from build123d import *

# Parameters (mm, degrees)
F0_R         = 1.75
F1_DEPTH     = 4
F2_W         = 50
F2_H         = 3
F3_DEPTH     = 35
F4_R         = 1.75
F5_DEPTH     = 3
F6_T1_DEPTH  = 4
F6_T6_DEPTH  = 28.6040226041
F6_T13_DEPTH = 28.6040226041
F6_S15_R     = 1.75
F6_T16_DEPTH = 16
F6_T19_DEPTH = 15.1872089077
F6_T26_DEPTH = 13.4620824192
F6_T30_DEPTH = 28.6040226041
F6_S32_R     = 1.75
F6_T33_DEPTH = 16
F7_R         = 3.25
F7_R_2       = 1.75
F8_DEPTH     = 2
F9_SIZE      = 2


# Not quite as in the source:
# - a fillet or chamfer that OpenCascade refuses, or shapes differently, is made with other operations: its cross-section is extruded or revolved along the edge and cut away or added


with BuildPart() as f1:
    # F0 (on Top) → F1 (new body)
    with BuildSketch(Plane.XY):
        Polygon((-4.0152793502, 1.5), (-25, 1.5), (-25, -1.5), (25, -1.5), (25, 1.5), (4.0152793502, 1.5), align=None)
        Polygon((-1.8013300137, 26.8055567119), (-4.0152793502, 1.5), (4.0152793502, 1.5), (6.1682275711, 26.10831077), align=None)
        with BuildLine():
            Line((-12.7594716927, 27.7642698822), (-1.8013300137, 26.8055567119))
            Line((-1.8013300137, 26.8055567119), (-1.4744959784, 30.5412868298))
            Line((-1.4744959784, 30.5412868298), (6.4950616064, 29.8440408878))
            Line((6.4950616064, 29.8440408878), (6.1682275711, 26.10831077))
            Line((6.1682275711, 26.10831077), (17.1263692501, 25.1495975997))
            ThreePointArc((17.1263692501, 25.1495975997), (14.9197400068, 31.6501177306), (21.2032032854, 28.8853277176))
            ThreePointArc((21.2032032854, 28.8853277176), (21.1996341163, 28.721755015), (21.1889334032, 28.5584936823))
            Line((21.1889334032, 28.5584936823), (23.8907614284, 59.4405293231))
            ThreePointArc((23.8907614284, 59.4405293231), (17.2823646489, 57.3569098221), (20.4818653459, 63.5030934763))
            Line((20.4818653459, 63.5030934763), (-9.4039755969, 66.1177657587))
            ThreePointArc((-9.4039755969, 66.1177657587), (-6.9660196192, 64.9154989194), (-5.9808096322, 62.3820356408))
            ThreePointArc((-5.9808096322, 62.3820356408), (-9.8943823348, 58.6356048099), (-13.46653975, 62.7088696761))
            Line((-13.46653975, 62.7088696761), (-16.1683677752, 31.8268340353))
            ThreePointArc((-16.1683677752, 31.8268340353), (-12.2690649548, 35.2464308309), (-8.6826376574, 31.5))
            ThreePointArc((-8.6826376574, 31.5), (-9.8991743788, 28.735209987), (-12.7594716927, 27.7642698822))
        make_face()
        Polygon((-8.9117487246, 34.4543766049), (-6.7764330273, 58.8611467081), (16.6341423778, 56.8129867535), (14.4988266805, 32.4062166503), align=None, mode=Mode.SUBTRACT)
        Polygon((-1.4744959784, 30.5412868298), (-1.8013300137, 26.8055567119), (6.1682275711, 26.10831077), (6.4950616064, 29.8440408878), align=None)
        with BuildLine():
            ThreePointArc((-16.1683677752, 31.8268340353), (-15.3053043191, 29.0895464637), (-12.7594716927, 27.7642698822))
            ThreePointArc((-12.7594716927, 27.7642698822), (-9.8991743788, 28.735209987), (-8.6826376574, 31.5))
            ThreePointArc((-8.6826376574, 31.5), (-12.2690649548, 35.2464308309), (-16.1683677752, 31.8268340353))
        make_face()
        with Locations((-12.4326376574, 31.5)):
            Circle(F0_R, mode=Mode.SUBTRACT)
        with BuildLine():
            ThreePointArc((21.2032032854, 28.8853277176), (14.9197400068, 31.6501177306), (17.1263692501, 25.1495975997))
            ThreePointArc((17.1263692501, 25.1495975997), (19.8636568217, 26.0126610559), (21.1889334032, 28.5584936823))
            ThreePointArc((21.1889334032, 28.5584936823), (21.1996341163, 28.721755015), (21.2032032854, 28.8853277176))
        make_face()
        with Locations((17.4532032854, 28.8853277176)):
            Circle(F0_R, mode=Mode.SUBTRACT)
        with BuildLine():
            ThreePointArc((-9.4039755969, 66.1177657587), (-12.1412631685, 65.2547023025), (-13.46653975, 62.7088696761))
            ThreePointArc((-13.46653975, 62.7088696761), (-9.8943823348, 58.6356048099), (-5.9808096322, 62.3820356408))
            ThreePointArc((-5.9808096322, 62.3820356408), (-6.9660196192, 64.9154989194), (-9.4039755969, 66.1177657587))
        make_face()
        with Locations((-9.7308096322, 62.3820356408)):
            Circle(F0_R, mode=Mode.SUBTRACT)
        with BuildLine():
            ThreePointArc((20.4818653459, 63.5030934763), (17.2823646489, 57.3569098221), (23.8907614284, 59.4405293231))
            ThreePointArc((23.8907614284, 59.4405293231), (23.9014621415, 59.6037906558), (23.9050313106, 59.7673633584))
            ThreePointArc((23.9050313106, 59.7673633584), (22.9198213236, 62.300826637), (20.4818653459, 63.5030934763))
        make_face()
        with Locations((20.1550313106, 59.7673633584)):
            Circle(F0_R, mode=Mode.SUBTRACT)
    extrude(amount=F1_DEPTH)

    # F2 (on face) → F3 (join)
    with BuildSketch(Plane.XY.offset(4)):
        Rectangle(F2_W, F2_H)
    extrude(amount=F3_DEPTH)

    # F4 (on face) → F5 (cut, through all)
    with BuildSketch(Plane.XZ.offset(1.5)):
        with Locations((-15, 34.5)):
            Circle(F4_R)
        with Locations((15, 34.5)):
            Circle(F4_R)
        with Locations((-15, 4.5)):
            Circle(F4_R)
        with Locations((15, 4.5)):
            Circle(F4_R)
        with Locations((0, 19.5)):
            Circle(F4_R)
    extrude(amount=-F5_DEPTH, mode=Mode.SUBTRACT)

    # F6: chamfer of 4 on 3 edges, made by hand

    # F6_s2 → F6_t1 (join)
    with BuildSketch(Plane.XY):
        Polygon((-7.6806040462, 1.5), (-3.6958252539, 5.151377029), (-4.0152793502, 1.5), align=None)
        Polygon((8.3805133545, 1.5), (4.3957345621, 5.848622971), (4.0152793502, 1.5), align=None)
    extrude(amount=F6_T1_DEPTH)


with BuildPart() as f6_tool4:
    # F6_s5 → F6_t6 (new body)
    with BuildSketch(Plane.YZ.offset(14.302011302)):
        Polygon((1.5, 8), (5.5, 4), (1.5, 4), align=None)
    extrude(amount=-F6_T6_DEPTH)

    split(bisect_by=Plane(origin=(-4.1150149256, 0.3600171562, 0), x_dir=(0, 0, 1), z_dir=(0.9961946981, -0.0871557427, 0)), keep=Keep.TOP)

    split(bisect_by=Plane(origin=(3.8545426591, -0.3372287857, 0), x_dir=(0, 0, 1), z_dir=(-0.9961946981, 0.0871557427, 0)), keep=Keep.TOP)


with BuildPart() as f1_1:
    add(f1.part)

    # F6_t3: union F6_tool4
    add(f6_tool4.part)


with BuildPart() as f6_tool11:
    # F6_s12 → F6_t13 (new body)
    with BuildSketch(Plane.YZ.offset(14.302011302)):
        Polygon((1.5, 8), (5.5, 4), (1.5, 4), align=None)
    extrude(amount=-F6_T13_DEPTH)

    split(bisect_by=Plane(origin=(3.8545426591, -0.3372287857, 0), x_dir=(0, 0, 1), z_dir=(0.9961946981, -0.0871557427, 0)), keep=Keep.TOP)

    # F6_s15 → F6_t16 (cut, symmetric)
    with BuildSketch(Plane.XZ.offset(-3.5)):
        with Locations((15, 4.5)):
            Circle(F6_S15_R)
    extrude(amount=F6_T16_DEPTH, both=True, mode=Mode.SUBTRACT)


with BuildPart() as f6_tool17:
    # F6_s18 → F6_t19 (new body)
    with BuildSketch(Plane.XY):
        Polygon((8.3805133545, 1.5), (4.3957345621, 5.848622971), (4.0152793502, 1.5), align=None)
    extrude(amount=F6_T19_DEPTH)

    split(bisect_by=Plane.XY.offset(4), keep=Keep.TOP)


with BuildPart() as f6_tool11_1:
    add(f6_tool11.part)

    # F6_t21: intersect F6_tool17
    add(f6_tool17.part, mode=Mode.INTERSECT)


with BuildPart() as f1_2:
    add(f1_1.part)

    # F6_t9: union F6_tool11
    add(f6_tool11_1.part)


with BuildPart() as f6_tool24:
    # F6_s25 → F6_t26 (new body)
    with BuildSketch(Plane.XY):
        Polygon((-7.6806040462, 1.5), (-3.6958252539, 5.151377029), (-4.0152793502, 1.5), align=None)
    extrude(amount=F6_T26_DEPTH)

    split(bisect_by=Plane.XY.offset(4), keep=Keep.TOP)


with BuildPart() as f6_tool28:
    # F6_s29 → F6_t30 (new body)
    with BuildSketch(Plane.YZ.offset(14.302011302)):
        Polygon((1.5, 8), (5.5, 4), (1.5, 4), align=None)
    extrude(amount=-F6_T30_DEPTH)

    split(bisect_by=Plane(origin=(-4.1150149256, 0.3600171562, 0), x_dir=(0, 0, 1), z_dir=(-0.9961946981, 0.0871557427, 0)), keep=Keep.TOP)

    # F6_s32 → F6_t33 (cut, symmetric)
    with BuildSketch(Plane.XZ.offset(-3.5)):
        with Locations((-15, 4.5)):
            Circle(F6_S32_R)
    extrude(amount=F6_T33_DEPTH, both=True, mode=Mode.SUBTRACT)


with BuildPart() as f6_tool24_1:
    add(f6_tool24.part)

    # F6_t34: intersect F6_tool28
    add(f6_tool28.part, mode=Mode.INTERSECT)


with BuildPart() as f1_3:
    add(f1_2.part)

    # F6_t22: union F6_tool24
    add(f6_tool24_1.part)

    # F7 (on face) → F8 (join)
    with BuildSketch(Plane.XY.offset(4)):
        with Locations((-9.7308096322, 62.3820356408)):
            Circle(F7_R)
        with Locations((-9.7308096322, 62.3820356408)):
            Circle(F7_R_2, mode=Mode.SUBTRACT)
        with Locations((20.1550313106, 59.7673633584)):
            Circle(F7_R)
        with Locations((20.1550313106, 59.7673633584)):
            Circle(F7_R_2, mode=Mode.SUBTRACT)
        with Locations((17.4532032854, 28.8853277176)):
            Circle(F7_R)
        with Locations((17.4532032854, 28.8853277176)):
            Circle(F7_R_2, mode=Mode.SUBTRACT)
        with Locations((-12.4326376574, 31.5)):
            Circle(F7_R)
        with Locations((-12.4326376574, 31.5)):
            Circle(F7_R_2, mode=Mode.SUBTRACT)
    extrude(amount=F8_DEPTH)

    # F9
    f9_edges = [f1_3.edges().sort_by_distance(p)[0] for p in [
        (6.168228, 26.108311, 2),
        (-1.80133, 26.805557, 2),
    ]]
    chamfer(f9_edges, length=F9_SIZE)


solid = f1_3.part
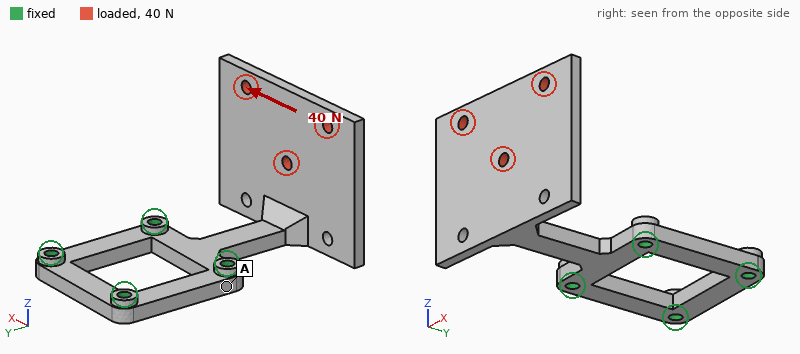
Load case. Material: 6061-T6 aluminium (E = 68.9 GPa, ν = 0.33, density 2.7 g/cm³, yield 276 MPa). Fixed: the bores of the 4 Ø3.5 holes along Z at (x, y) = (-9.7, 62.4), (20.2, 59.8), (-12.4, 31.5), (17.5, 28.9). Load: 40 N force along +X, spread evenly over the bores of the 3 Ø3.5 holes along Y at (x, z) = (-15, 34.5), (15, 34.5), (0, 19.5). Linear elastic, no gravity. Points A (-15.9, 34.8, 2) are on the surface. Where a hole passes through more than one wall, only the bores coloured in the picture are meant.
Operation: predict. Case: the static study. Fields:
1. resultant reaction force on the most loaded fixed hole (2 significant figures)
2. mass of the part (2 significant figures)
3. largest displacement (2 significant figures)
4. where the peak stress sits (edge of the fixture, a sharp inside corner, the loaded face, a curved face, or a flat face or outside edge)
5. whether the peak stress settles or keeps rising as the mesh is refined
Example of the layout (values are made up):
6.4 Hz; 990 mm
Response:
81 N; 27 g; 0.42 mm; a sharp inside corner; keeps rising
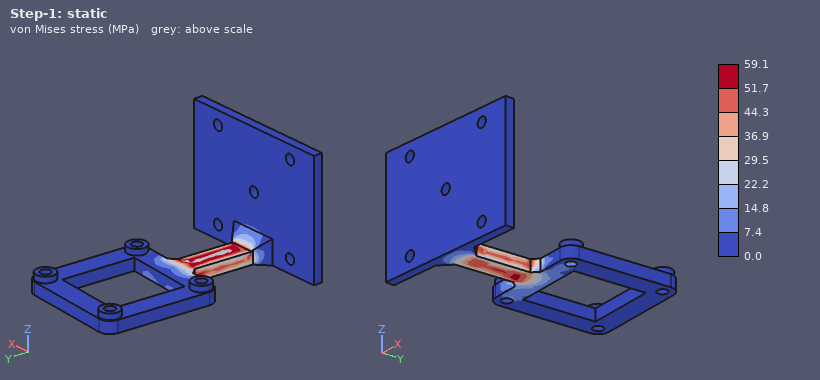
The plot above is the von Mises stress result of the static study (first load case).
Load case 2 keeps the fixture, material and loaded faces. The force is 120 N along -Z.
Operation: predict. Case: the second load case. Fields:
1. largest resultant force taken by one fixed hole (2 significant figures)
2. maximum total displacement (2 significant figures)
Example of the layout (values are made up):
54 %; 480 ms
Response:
66 N; 1.0 mm
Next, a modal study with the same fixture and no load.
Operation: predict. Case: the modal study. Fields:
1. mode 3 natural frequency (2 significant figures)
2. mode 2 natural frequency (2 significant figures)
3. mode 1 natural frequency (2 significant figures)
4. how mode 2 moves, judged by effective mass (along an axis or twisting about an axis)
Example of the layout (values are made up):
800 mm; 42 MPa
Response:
1300 Hz; 560 Hz; 440 Hz; along X
